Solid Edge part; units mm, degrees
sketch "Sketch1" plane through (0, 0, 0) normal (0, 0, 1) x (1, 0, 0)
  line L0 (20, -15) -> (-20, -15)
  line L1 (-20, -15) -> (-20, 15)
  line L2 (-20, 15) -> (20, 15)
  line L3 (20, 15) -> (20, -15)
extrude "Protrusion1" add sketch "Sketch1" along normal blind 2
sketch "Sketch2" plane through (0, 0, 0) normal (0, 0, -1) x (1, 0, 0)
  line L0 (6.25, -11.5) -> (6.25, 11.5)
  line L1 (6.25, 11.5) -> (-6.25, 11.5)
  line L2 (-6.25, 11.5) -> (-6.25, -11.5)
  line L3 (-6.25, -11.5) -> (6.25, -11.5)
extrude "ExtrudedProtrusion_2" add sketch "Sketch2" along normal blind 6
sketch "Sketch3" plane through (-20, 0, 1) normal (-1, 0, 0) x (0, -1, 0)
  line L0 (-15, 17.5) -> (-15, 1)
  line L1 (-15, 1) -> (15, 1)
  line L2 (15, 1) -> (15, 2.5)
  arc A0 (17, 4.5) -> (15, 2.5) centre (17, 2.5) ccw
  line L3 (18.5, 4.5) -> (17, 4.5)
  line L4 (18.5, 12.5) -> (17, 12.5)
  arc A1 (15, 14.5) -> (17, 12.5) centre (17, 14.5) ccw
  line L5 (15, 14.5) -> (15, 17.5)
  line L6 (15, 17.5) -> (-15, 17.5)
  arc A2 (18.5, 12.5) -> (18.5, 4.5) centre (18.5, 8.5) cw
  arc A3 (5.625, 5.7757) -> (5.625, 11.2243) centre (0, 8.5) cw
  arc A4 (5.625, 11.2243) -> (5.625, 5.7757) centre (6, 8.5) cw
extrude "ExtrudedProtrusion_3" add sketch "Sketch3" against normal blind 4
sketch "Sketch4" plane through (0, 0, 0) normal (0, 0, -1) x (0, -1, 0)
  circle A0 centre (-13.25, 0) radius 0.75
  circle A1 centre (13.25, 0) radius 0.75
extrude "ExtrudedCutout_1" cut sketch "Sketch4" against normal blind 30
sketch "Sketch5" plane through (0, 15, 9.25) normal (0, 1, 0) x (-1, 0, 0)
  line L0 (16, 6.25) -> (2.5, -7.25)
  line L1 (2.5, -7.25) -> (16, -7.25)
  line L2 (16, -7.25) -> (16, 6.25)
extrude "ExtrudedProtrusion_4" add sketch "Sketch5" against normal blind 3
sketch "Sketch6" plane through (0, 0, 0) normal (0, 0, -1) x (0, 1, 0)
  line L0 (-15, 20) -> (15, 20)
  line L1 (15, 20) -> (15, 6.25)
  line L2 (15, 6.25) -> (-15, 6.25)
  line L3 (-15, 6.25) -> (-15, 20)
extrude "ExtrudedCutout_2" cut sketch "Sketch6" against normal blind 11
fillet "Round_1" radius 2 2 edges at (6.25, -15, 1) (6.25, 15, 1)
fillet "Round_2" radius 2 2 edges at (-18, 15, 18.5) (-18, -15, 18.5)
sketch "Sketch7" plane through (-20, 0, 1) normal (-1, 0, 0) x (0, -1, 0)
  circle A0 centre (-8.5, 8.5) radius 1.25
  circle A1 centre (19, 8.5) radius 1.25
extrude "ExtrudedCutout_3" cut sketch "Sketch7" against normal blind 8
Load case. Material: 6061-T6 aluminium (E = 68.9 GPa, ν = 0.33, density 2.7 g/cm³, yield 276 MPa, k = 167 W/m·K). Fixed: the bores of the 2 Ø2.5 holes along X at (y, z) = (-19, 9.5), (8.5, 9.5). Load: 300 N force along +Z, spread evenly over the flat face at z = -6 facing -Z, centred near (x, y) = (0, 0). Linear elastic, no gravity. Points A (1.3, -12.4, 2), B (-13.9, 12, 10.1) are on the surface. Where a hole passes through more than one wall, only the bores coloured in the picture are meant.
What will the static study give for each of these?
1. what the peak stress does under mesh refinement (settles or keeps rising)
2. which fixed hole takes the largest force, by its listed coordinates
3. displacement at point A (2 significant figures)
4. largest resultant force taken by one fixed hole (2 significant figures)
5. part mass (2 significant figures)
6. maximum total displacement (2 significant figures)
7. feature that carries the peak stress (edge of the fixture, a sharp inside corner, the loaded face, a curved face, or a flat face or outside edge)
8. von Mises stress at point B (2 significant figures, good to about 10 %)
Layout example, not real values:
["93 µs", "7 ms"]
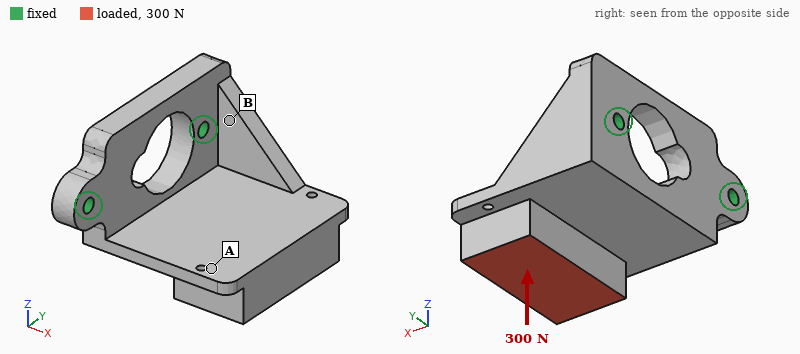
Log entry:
["keeps rising", "(8.5, 9.5)", "0.22 mm", "190 N", "14 g", "0.30 mm", "edge of the fixture", "45 MPa"]
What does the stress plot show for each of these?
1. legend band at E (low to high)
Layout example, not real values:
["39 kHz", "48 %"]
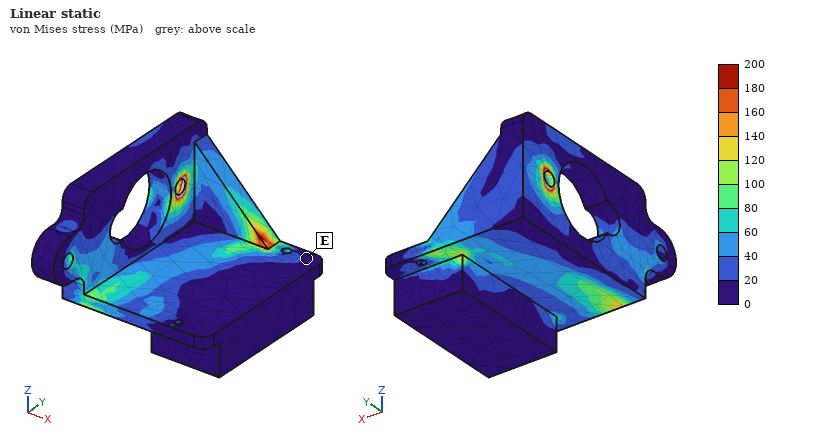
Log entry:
["0 to 20 MPa"]
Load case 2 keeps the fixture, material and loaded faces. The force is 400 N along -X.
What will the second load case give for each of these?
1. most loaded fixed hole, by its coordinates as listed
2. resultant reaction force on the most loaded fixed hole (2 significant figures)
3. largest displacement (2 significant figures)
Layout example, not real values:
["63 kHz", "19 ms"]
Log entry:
["(8.5, 9.5)", "270 N", "0.26 mm"]
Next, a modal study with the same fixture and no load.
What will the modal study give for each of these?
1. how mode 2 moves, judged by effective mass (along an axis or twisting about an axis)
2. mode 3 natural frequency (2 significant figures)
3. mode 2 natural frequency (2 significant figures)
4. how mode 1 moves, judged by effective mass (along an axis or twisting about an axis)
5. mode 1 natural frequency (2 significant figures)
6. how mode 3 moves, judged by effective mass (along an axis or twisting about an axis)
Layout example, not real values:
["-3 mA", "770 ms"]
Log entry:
["along Y", "7800 Hz", "5700 Hz", "along Z", "2300 Hz", "along X"]
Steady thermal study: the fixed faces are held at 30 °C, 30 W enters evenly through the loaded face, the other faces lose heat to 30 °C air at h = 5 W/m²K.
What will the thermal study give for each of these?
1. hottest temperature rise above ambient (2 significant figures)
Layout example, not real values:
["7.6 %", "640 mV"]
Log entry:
["59 K"]
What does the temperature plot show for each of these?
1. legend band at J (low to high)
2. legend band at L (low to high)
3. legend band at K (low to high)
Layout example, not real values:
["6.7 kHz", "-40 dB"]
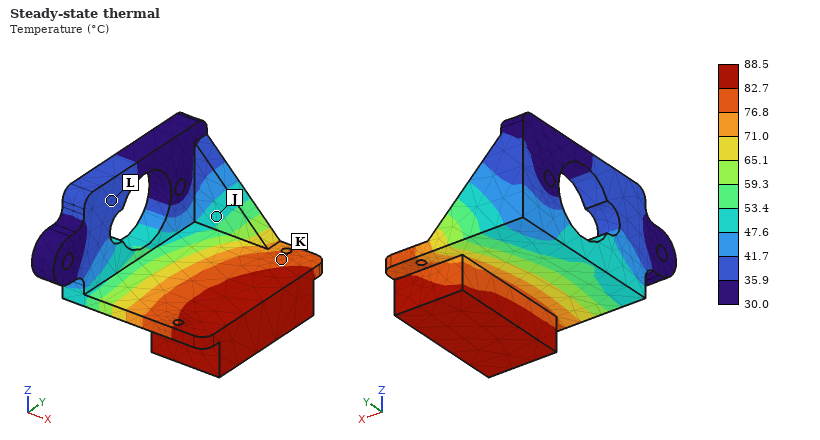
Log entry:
["47.6 to 53.4 °C", "35.9 to 41.7 °C", "76.8 to 82.7 °C"]
